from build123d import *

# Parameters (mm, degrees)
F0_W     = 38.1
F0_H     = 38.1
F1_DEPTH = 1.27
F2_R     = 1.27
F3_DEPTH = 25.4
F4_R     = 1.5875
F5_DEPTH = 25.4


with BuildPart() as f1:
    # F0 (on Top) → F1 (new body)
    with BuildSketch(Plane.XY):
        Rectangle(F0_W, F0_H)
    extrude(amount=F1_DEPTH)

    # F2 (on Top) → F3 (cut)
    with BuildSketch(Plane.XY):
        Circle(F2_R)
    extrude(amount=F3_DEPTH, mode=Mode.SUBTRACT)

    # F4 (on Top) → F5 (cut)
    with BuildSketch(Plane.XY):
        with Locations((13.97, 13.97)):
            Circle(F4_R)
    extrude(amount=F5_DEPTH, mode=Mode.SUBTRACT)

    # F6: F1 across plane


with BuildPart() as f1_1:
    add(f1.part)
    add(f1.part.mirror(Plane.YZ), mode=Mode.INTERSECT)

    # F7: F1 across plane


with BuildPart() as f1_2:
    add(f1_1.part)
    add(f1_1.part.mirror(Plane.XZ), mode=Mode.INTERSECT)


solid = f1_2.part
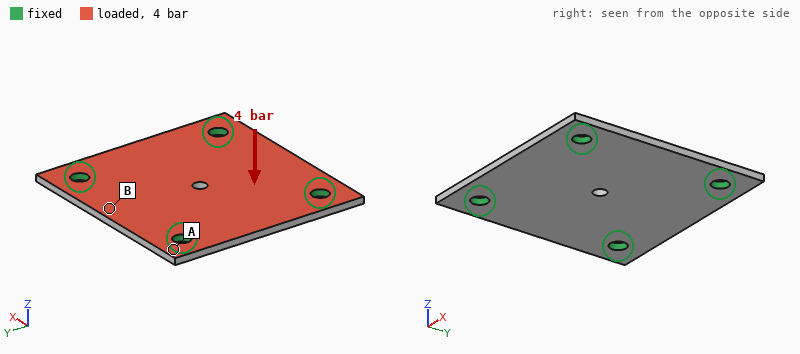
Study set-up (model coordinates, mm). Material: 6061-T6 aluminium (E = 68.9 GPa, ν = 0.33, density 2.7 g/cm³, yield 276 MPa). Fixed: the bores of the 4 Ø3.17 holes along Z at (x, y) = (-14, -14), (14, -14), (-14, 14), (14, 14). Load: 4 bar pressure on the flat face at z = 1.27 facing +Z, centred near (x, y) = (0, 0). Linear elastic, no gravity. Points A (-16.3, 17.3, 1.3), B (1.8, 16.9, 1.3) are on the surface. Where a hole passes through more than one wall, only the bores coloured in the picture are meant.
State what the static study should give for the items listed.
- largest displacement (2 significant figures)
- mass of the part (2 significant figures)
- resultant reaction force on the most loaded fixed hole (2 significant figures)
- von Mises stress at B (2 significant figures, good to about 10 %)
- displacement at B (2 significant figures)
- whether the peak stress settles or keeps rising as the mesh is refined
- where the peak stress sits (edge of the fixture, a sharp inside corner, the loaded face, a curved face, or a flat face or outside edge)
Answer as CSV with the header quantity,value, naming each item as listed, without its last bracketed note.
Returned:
quantity,value
largest displacement,0.10 mm
mass of the part,4.9 g
resultant reaction force on the most loaded fixed hole,140 N
von Mises stress at B,45 MPa
displacement at B,0.043 mm
whether the peak stress settles or keeps rising as the mesh is refined,keeps rising
where the peak stress sits,edge of the fixture
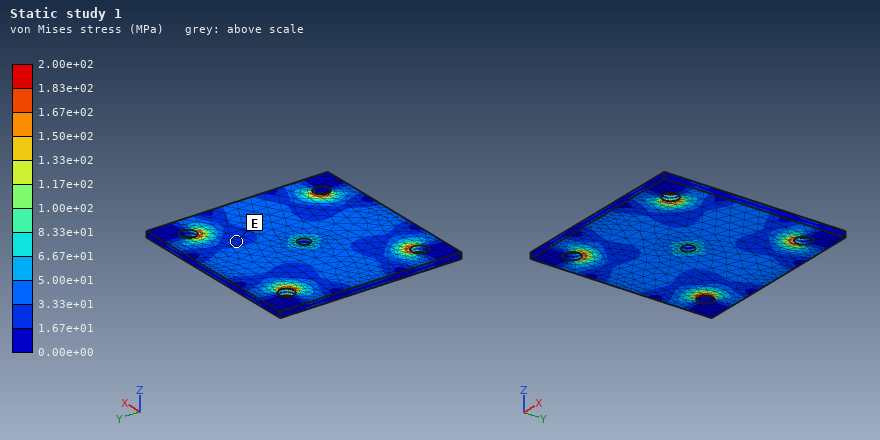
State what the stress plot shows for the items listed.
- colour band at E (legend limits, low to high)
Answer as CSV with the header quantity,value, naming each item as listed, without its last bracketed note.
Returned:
quantity,value
colour band at E,1.67e+01 to 3.33e+01 MPa
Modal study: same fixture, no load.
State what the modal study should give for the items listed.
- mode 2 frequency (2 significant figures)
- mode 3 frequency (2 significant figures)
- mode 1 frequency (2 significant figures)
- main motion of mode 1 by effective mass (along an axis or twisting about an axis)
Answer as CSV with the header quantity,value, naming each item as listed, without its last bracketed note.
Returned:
quantity,value
mode 2 frequency,10 kHz
mode 3 frequency,10 kHz
mode 1 frequency,6700 Hz
main motion of mode 1 by effective mass,along Z
